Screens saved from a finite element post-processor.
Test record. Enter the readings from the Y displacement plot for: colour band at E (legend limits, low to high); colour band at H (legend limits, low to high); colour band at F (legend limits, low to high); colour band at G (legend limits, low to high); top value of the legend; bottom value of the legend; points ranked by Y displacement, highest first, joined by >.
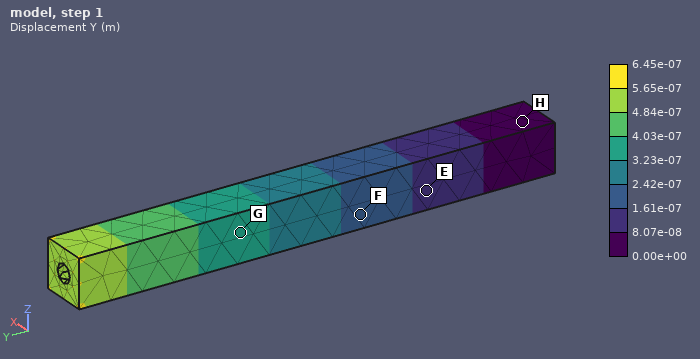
8.07e-08 to 1.61e-07 m
0.00e+00 to 8.07e-08 m
1.61e-07 to 2.42e-07 m
3.23e-07 to 4.03e-07 m
6.45e-07 m
0.00e+00 m
G > F > E > H
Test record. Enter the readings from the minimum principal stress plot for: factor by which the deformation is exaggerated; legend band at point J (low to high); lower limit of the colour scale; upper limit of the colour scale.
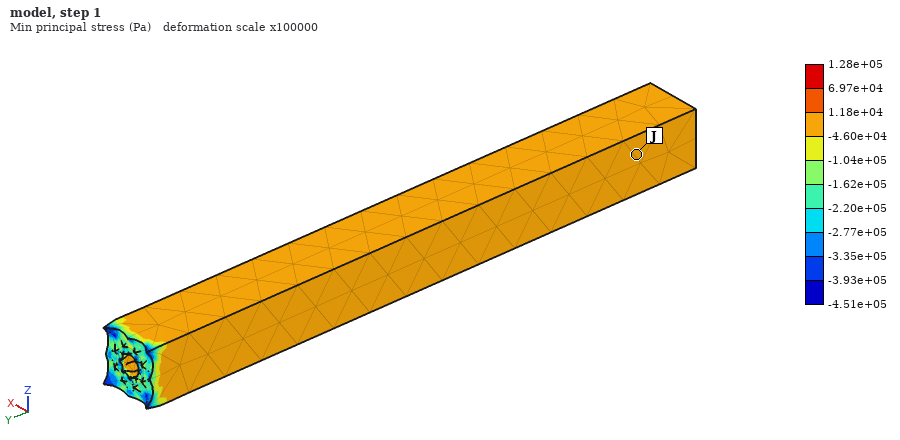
100000
-4.60e+04 to 1.18e+04 Pa
-4.51e+05 Pa
1.28e+05 Pa
